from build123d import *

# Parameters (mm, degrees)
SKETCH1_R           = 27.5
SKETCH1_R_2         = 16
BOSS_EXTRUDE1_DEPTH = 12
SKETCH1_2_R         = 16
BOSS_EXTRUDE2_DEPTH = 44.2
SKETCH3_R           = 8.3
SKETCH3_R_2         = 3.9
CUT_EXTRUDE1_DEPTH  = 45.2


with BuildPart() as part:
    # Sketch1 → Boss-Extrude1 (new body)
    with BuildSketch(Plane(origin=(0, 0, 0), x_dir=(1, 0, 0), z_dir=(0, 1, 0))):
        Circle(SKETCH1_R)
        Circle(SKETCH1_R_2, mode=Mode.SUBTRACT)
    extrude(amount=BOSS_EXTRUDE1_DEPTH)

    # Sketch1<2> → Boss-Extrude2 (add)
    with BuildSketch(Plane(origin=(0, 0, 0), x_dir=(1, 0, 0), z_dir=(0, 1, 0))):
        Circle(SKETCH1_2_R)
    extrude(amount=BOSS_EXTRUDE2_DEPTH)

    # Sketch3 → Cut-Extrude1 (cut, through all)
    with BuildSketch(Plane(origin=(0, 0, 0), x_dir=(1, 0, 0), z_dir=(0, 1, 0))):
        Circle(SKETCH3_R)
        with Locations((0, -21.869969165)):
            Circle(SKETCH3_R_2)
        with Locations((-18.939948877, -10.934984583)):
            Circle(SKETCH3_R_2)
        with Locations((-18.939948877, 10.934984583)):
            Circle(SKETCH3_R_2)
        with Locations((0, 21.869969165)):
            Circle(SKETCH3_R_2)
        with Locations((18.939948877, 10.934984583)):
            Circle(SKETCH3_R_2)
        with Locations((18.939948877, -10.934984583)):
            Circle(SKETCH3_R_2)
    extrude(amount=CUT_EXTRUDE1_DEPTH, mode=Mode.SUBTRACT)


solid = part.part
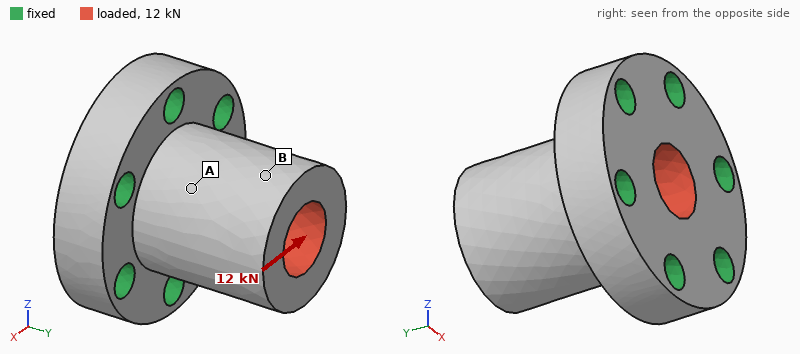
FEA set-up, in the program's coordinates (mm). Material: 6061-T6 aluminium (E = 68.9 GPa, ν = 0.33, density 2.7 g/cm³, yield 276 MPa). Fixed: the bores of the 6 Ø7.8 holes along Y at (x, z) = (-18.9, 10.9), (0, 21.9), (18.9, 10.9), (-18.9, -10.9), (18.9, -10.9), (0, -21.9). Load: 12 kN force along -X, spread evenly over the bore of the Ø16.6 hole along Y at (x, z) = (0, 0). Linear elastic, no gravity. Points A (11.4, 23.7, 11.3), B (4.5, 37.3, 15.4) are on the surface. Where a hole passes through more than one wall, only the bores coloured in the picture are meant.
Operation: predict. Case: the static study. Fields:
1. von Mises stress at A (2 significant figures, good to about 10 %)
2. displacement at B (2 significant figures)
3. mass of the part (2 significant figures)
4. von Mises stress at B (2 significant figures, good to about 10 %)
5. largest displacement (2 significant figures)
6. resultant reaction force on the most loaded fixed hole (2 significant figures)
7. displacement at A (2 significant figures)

19 MPa
30 µm
110 g
8.3 MPa
40 µm
3.9 kN
18 µm
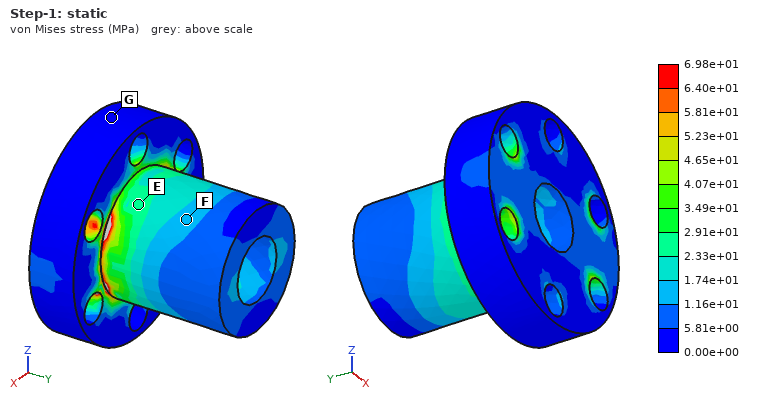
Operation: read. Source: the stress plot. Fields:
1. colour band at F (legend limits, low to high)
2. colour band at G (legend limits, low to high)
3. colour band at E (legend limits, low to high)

1.16e+01 to 1.74e+01 MPa
0.00e+00 to 5.81e+00 MPa
2.33e+01 to 2.91e+01 MPa
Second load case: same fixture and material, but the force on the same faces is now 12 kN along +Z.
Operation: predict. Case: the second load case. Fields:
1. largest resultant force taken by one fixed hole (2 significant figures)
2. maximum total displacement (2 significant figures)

4.4 kN
40 µm
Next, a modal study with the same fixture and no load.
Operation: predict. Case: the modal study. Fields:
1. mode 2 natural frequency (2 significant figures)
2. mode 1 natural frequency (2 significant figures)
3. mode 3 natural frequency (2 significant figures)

12 kHz
12 kHz
22 kHz
